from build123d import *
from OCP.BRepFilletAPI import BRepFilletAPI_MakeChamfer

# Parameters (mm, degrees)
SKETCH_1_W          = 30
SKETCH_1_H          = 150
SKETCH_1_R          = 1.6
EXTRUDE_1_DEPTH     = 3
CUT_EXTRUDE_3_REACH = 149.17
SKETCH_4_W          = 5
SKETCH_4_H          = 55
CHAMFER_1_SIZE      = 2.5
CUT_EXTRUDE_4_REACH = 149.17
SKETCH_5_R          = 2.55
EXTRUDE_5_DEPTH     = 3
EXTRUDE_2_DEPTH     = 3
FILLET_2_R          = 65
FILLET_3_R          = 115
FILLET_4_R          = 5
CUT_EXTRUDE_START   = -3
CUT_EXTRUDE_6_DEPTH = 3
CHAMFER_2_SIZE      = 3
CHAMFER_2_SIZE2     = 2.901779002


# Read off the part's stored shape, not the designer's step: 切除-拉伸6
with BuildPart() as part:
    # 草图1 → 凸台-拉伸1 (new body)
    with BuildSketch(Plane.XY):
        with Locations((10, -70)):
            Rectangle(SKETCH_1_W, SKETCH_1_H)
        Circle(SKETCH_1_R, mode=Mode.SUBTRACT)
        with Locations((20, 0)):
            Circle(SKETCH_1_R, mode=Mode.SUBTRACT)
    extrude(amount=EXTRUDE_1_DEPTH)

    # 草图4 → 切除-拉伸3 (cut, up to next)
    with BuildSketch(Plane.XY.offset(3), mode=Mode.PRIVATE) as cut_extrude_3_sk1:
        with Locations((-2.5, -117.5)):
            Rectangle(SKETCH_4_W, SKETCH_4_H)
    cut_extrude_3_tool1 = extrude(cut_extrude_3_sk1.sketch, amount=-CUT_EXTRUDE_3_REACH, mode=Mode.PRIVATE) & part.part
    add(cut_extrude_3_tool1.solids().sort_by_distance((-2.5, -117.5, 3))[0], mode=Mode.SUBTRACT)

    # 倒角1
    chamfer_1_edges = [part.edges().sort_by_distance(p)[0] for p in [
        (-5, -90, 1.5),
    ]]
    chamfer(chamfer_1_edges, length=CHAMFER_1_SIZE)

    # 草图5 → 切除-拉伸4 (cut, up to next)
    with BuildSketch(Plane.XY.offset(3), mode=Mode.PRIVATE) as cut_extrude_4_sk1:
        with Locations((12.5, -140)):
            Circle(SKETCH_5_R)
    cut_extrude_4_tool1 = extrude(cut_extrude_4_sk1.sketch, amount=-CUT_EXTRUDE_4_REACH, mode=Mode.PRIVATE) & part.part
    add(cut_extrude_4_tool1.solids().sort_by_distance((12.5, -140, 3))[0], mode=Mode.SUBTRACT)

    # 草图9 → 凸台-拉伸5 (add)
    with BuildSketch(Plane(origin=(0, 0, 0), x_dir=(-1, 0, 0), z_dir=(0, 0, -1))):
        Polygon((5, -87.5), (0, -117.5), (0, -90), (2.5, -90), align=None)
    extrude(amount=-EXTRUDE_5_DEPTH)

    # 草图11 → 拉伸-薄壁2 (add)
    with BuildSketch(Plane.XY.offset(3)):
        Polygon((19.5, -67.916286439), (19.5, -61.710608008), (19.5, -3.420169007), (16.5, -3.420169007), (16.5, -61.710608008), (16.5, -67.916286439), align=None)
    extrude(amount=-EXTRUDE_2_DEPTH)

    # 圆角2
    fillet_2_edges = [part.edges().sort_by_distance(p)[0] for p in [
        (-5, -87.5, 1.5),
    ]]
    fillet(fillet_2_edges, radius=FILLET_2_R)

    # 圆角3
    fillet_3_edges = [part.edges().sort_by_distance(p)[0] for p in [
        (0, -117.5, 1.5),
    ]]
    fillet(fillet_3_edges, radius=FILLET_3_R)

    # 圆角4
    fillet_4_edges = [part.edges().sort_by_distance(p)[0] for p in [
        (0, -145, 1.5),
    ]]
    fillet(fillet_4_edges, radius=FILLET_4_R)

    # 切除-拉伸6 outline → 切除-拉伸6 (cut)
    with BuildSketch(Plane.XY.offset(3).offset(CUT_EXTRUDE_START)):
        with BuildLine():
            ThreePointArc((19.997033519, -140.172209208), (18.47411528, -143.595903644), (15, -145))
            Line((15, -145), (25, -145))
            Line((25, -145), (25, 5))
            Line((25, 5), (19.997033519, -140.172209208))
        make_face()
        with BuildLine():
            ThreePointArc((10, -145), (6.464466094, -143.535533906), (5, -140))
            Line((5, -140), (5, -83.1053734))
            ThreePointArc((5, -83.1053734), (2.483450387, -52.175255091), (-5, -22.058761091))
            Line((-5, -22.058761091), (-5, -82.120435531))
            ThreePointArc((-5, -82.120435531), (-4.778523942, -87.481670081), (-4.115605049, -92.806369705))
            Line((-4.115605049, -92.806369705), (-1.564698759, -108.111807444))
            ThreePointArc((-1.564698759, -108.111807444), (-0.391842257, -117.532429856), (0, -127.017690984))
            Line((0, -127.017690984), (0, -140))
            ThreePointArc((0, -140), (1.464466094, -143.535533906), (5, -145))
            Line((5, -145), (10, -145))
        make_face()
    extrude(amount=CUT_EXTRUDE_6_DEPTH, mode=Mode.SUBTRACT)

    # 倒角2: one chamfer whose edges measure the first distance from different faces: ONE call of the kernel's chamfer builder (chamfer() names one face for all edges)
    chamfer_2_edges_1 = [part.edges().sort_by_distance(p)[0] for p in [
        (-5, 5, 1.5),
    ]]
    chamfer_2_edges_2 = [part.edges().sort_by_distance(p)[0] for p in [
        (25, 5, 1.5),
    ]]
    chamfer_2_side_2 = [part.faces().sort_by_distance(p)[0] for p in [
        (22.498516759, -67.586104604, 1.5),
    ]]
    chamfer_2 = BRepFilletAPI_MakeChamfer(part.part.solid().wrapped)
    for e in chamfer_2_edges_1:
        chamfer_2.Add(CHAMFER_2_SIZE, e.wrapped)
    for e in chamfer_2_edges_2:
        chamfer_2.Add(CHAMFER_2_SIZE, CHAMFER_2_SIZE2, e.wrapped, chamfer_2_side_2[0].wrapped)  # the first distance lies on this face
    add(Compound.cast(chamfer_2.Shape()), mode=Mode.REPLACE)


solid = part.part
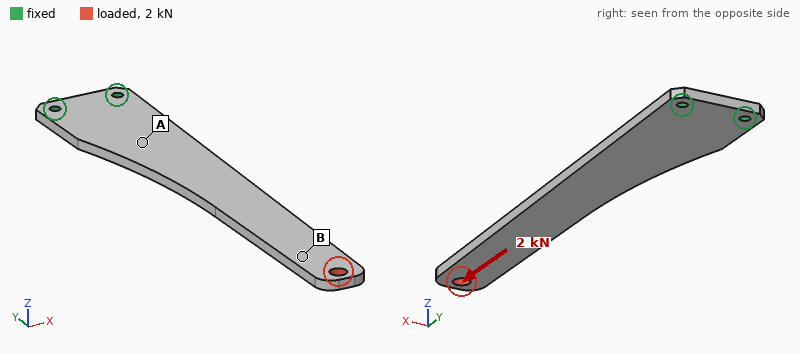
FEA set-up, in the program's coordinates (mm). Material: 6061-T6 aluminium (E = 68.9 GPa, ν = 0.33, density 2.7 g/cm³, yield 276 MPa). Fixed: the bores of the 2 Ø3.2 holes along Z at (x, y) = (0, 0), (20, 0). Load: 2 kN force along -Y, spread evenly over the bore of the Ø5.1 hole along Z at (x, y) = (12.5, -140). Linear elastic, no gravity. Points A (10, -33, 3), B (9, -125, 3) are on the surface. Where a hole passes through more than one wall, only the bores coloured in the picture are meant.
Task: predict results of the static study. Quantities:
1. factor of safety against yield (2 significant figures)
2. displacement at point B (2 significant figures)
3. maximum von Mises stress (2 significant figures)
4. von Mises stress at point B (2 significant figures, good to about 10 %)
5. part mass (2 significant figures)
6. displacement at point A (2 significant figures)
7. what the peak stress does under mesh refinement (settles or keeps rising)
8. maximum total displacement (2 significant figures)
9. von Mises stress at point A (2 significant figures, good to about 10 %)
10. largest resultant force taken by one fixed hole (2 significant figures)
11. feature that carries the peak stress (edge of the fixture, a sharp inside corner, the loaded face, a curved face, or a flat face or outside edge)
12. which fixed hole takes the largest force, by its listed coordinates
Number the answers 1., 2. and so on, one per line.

1. 1.9
2. 67 µm
3. 140 MPa
4. 45 MPa
5. 25 g
6. 14 µm
7. settles
8. 83 µm
9. 26 MPa
10. 1.2 kN
11. the loaded face
12. (20, 0)
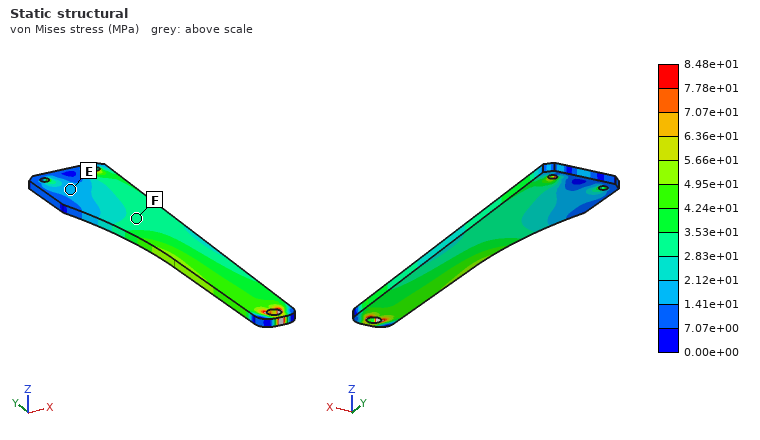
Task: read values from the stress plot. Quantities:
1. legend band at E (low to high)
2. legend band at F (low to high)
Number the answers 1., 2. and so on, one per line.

1. 1.41e+01 to 2.12e+01 MPa
2. 2.83e+01 to 3.53e+01 MPa
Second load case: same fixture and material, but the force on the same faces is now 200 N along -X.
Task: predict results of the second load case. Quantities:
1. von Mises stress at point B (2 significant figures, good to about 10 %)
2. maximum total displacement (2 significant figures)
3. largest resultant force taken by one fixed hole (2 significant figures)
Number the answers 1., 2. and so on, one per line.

1. 14 MPa
2. 0.99 mm
3. 1.3 kN
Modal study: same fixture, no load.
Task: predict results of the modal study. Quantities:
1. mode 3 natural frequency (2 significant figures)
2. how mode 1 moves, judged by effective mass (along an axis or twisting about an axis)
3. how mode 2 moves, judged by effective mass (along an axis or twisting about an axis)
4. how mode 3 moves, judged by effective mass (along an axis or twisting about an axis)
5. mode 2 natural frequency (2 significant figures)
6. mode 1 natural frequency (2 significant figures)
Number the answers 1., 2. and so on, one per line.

1. 1200 Hz
2. along Z
3. along Z
4. along X
5. 800 Hz
6. 150 Hz
